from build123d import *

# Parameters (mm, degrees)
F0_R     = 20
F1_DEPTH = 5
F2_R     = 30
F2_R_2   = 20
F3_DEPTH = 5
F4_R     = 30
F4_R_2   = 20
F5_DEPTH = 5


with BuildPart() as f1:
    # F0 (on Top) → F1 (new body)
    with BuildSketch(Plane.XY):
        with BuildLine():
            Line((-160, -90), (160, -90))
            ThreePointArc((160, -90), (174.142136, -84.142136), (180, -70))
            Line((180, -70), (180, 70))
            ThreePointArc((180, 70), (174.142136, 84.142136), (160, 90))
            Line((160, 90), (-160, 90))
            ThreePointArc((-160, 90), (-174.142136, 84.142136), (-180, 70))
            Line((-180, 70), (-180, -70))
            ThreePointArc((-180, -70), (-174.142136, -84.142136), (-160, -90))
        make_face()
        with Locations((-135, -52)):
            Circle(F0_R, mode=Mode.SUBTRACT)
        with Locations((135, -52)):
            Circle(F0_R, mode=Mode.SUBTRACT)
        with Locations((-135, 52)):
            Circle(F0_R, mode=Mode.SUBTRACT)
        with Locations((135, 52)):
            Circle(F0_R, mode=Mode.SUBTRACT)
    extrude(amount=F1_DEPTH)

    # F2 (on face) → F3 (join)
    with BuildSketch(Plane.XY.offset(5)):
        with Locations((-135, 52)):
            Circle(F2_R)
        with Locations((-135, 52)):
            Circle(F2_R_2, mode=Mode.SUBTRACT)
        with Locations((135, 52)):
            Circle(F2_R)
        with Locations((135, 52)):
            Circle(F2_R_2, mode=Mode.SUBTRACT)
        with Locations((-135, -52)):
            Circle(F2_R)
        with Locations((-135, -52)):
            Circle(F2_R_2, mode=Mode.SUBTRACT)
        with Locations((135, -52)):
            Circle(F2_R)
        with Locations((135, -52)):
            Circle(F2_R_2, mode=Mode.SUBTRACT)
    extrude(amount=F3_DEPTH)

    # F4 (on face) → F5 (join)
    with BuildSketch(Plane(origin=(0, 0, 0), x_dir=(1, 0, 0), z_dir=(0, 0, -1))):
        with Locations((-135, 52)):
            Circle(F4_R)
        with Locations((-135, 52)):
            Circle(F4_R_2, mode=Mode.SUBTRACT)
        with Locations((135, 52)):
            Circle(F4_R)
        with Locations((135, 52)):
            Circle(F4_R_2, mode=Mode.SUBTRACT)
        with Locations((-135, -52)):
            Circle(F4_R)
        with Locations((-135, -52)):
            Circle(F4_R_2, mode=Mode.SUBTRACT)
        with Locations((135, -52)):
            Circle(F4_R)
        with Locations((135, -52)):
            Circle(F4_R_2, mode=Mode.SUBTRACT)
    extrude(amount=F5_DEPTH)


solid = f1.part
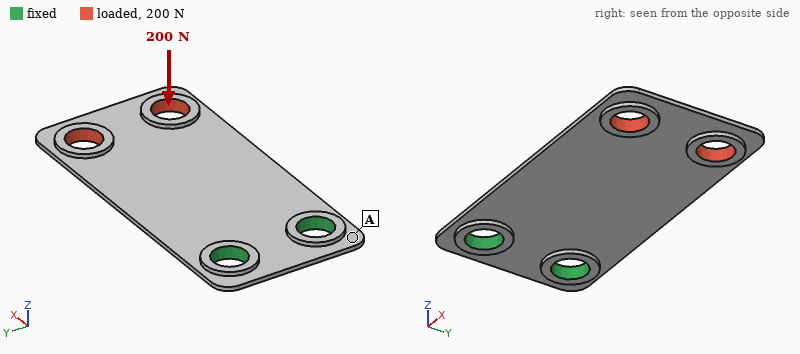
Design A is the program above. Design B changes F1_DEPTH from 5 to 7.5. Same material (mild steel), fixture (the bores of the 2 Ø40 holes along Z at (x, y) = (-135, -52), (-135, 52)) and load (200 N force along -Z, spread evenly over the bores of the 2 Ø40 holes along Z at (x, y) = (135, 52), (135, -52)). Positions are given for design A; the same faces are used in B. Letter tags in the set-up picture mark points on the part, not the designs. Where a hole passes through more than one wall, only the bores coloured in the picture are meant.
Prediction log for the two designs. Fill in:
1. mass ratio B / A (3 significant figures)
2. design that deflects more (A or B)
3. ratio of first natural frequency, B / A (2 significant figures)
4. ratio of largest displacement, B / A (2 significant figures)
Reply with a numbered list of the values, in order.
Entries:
1. 1.37
2. A
3. 1.6
4. 0.30
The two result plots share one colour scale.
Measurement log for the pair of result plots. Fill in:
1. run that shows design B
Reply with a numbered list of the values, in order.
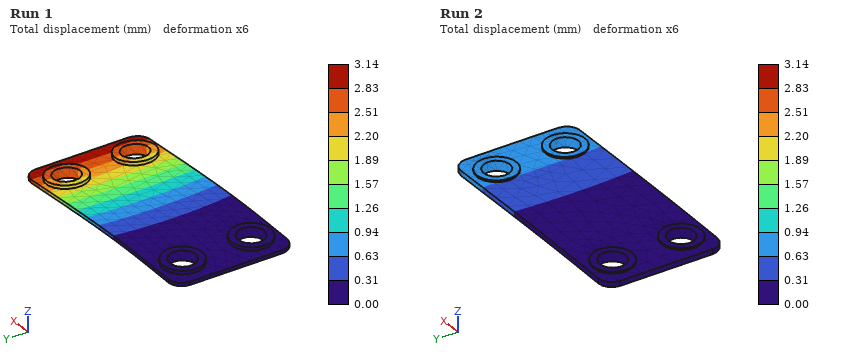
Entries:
1. Run 2
